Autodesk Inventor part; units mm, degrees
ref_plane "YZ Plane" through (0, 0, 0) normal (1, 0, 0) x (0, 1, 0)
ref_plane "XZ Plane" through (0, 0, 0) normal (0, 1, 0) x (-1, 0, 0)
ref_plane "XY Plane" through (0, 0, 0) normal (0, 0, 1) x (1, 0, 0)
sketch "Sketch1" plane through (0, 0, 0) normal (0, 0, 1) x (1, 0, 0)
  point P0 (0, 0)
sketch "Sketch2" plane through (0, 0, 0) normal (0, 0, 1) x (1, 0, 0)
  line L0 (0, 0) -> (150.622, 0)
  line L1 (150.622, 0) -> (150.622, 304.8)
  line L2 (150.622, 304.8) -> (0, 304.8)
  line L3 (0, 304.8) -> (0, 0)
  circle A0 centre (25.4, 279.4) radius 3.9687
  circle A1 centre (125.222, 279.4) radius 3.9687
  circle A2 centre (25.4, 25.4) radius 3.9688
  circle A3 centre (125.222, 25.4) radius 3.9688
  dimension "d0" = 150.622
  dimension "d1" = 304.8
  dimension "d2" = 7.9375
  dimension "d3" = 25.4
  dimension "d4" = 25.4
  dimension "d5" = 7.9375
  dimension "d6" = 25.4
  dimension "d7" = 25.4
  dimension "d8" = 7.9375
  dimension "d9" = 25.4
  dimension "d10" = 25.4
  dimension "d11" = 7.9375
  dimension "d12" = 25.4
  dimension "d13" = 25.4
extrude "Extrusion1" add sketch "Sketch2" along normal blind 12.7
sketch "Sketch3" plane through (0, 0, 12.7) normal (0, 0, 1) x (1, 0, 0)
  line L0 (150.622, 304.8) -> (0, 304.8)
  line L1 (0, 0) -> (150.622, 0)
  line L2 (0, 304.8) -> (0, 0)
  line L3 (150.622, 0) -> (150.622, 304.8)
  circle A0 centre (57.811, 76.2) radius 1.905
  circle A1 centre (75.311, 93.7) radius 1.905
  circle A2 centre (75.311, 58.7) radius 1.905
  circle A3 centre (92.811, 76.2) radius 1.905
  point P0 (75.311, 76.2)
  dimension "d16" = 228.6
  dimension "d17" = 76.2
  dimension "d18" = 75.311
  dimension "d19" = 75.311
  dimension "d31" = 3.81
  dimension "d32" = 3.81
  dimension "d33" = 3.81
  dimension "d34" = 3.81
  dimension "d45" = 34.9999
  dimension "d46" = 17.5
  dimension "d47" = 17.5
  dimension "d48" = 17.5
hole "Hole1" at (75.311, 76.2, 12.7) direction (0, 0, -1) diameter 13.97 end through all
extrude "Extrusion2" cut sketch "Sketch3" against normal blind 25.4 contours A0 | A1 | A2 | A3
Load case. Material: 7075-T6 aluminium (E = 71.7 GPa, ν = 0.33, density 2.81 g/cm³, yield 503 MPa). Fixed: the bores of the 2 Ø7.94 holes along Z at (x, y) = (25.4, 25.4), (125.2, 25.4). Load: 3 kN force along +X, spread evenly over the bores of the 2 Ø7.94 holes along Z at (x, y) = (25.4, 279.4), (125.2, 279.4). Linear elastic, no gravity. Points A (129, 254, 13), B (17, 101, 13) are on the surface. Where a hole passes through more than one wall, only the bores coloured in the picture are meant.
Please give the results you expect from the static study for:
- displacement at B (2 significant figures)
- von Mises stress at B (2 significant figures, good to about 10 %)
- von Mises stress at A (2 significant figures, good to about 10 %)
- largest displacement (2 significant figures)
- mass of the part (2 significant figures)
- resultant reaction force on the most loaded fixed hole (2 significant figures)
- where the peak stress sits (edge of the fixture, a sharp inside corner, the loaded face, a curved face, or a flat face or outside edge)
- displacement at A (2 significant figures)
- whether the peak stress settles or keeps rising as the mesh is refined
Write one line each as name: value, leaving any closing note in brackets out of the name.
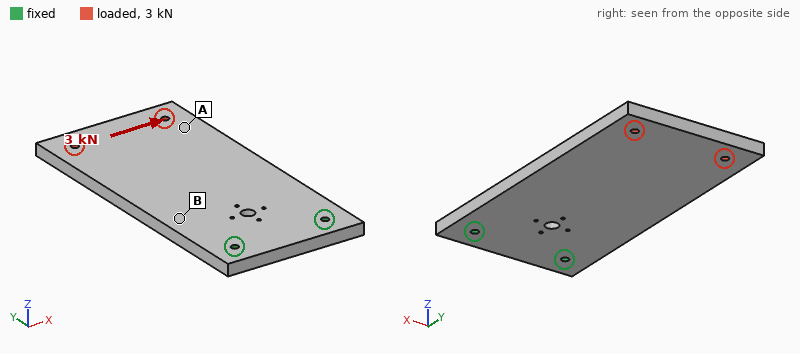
displacement at B: 0.024 mm
von Mises stress at B: 8.6 MPa
von Mises stress at A: 2.6 MPa
largest displacement: 0.11 mm
mass of the part: 1.6 kg
resultant reaction force on the most loaded fixed hole: 7.6 kN
where the peak stress sits: edge of the fixture
displacement at A: 0.087 mm
whether the peak stress settles or keeps rising as the mesh is refined: keeps rising
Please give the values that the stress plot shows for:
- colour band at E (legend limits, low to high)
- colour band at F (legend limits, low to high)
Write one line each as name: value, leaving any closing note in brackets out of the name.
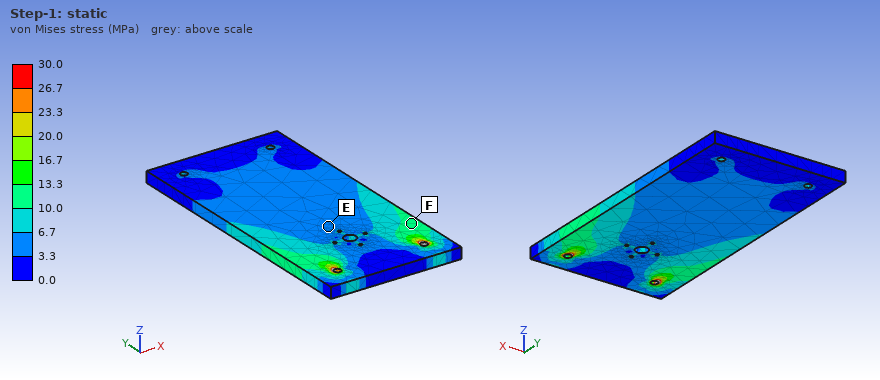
colour band at E: 3.3 to 6.7 MPa
colour band at F: 10.0 to 13.3 MPa
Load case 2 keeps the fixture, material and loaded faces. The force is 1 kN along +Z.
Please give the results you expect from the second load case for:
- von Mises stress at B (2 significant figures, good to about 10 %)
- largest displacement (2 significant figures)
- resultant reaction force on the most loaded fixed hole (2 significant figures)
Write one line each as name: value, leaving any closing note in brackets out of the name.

von Mises stress at B: 45 MPa
largest displacement: 3.8 mm
resultant reaction force on the most loaded fixed hole: 500 N
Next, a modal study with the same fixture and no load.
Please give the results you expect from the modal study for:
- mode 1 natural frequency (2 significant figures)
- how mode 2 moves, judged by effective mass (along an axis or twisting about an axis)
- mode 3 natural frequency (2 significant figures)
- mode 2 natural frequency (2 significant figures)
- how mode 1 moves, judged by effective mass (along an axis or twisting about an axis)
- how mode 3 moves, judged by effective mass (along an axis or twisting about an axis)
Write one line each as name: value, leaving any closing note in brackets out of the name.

mode 1 natural frequency: 120 Hz
how mode 2 moves, judged by effective mass: twisting about Y
mode 3 natural frequency: 790 Hz
mode 2 natural frequency: 520 Hz
how mode 1 moves, judged by effective mass: along Z
how mode 3 moves, judged by effective mass: along Z
